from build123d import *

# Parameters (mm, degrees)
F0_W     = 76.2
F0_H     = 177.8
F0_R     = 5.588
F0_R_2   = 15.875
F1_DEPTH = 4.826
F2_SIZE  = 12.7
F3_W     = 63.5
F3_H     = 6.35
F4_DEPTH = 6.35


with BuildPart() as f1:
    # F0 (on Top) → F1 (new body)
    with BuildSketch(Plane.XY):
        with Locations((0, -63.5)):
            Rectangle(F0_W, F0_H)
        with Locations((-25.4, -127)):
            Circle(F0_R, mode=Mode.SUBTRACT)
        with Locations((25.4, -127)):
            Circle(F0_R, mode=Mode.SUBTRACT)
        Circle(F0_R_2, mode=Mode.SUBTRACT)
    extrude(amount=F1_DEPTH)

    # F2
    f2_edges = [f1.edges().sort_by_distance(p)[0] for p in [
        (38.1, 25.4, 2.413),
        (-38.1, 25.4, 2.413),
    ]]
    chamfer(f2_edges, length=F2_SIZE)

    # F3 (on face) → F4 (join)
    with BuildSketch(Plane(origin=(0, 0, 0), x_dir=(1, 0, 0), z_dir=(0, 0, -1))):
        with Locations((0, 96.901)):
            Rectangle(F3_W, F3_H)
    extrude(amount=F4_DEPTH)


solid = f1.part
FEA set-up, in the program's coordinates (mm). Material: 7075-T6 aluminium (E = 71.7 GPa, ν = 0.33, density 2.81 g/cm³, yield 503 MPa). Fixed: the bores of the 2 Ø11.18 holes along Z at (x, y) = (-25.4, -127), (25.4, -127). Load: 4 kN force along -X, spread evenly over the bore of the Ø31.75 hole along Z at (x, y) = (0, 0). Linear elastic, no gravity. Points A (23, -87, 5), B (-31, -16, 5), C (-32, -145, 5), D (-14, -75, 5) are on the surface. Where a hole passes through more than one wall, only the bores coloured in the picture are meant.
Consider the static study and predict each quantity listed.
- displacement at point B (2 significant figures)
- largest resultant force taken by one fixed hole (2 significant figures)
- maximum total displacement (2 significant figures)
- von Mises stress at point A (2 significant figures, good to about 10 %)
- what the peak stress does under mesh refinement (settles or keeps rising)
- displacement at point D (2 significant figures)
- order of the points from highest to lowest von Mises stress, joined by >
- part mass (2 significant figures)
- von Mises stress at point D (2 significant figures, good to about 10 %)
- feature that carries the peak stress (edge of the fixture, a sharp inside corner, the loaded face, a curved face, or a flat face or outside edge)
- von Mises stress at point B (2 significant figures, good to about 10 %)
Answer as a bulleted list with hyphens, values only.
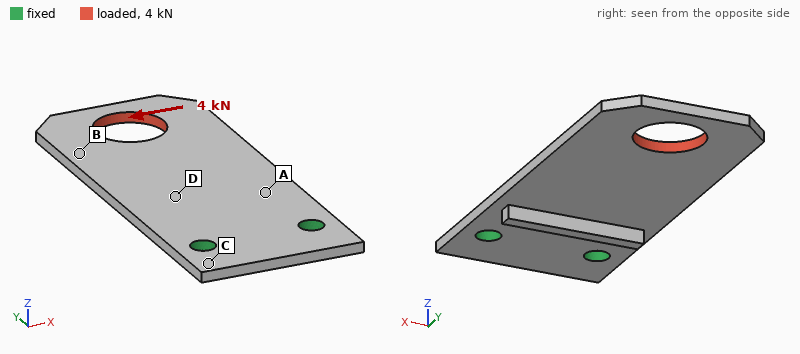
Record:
- 0.24 mm
- 9.3 kN
- 0.37 mm
- 48 MPa
- keeps rising
- 0.071 mm
- A > D > B > C
- 180 g
- 35 MPa
- edge of the fixture
- 21 MPa
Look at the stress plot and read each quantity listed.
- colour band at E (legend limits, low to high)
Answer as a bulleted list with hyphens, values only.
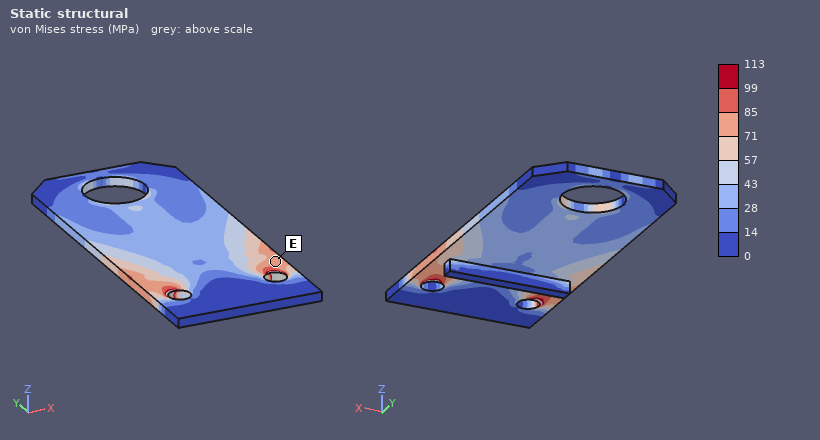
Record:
- 71 to 85 MPa
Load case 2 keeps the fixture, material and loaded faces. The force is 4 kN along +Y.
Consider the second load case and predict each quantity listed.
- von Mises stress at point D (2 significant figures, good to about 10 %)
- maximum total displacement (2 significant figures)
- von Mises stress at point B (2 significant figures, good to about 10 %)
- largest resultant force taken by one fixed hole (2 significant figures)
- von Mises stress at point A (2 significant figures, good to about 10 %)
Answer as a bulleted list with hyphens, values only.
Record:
- 11 MPa
- 39 µm
- 11 MPa
- 2.0 kN
- 11 MPa
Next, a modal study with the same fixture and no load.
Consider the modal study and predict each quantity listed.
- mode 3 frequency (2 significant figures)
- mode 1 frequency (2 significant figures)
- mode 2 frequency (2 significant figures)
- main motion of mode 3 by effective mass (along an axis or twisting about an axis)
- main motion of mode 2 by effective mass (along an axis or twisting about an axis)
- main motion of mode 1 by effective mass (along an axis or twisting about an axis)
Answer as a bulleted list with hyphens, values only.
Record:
- 1100 Hz
- 210 Hz
- 800 Hz
- along Z
- twisting about Y
- along Z
